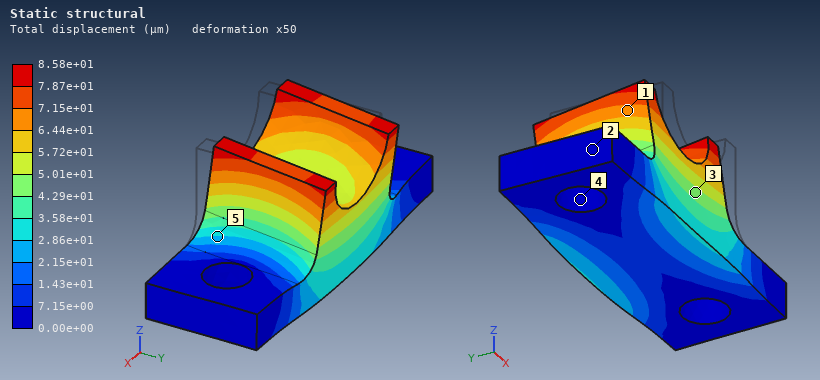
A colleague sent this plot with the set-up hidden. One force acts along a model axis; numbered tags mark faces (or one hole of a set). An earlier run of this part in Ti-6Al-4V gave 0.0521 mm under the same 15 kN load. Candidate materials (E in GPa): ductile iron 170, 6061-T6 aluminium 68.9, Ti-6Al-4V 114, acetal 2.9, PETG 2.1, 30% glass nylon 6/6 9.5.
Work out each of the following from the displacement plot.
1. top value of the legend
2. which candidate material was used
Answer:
8.58e+01 µm
6061-T6 aluminium
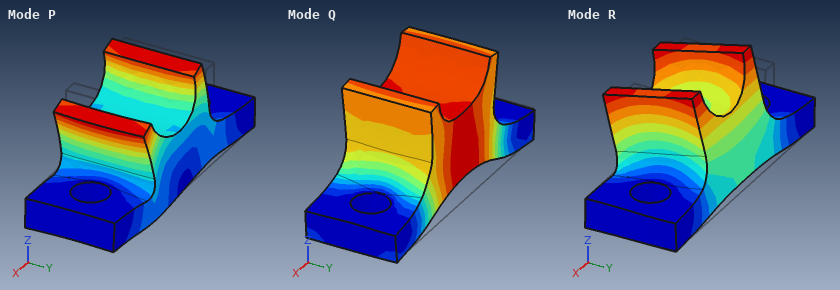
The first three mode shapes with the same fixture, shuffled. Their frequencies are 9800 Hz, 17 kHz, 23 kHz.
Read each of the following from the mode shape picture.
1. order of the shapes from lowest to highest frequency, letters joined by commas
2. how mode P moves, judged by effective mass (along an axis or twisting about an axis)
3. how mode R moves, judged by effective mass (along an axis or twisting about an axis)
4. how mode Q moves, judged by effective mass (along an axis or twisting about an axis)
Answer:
R, Q, P
along X
along Y
along Z
